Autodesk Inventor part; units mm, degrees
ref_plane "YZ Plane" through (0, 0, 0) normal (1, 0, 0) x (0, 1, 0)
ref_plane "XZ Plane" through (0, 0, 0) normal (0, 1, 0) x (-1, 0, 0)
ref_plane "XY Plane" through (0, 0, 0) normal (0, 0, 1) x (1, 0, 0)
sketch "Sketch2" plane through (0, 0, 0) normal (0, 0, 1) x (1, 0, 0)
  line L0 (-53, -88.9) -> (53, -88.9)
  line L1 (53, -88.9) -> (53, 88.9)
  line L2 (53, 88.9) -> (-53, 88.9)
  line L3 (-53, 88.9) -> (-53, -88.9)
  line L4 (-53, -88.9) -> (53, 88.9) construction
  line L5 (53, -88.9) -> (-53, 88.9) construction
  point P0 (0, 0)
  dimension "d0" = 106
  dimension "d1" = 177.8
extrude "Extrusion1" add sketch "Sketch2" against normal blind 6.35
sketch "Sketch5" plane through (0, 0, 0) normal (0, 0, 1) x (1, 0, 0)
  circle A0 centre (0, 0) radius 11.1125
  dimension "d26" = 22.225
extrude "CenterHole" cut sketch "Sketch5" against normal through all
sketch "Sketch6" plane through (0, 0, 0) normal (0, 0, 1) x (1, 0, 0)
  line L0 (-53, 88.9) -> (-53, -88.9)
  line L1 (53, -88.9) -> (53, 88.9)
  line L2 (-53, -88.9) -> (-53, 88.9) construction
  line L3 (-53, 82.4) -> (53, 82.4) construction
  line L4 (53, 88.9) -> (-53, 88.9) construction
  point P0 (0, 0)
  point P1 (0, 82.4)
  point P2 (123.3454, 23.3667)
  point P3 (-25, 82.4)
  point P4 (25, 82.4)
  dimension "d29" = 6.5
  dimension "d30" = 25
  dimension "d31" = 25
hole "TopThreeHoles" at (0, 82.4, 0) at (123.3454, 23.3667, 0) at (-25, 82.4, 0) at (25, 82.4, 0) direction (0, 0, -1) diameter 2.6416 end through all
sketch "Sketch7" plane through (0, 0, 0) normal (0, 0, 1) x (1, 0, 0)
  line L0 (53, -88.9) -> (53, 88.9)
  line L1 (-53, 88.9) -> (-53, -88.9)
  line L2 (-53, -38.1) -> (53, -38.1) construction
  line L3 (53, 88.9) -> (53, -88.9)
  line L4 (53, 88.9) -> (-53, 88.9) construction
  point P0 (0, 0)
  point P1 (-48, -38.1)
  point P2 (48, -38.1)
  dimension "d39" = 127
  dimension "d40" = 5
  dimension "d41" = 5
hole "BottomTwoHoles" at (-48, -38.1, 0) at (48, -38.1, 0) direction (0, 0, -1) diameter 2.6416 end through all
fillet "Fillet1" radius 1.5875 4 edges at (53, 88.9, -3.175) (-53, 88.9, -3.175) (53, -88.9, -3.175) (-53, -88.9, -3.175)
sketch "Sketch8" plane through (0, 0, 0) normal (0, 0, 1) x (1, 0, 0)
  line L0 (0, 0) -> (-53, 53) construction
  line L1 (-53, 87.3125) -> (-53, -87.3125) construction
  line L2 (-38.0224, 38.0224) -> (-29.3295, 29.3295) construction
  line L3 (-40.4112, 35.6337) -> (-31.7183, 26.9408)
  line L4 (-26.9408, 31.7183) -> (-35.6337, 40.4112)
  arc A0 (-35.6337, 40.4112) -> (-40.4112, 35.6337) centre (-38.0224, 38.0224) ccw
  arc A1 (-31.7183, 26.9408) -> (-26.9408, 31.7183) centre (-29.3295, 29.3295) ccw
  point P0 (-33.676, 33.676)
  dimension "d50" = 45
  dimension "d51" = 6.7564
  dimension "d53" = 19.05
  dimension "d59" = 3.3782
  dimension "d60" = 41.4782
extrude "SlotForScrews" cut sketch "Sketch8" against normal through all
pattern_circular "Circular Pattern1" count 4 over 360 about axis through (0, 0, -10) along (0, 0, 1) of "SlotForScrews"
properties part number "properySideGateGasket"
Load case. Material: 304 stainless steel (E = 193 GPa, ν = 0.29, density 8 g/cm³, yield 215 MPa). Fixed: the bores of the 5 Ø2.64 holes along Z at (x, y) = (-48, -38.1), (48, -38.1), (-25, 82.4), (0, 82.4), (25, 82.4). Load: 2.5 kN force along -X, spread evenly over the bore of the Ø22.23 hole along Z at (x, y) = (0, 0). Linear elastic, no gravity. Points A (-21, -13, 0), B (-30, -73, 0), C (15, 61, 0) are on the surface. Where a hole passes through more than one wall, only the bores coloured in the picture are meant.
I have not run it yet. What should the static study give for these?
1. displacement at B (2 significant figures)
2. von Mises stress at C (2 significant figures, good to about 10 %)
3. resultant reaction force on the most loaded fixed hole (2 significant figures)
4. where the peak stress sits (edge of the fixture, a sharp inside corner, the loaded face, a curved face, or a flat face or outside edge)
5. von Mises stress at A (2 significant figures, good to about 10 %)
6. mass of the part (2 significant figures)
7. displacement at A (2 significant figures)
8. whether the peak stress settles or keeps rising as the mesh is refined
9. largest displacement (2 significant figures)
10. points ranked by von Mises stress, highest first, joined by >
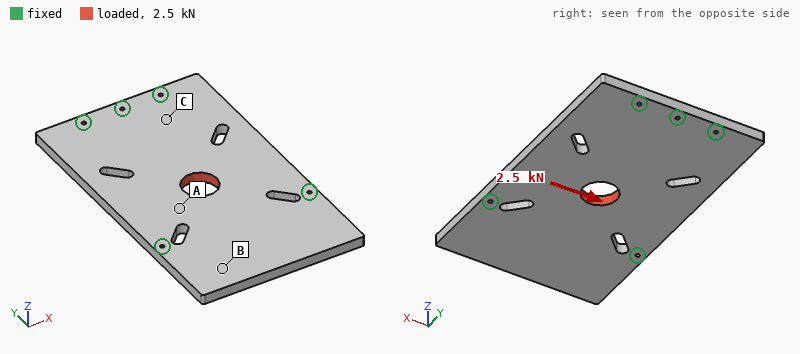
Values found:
1.0 µm
3.3 MPa
910 N
edge of the fixture
6.4 MPa
910 g
2.2 µm
keeps rising
3.0 µm
A > C > B
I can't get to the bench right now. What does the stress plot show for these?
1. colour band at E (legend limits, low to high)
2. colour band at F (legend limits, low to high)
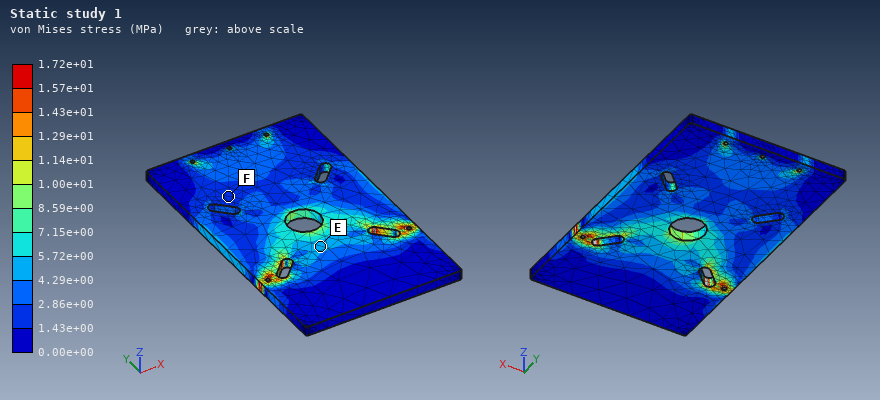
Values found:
4.29e+00 to 5.72e+00 MPa
1.43e+00 to 2.86e+00 MPa
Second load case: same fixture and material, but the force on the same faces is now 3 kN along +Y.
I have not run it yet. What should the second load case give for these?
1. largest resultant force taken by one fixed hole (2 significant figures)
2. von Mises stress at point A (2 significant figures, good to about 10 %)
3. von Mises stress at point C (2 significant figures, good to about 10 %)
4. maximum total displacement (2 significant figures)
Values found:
810 N
3.2 MPa
3.3 MPa
2.1 µm
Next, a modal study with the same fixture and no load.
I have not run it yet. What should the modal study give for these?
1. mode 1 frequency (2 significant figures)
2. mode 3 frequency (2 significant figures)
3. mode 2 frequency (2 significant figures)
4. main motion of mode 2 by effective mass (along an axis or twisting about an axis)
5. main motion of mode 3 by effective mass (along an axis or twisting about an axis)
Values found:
1100 Hz
2100 Hz
1600 Hz
along Z
twisting about Y
